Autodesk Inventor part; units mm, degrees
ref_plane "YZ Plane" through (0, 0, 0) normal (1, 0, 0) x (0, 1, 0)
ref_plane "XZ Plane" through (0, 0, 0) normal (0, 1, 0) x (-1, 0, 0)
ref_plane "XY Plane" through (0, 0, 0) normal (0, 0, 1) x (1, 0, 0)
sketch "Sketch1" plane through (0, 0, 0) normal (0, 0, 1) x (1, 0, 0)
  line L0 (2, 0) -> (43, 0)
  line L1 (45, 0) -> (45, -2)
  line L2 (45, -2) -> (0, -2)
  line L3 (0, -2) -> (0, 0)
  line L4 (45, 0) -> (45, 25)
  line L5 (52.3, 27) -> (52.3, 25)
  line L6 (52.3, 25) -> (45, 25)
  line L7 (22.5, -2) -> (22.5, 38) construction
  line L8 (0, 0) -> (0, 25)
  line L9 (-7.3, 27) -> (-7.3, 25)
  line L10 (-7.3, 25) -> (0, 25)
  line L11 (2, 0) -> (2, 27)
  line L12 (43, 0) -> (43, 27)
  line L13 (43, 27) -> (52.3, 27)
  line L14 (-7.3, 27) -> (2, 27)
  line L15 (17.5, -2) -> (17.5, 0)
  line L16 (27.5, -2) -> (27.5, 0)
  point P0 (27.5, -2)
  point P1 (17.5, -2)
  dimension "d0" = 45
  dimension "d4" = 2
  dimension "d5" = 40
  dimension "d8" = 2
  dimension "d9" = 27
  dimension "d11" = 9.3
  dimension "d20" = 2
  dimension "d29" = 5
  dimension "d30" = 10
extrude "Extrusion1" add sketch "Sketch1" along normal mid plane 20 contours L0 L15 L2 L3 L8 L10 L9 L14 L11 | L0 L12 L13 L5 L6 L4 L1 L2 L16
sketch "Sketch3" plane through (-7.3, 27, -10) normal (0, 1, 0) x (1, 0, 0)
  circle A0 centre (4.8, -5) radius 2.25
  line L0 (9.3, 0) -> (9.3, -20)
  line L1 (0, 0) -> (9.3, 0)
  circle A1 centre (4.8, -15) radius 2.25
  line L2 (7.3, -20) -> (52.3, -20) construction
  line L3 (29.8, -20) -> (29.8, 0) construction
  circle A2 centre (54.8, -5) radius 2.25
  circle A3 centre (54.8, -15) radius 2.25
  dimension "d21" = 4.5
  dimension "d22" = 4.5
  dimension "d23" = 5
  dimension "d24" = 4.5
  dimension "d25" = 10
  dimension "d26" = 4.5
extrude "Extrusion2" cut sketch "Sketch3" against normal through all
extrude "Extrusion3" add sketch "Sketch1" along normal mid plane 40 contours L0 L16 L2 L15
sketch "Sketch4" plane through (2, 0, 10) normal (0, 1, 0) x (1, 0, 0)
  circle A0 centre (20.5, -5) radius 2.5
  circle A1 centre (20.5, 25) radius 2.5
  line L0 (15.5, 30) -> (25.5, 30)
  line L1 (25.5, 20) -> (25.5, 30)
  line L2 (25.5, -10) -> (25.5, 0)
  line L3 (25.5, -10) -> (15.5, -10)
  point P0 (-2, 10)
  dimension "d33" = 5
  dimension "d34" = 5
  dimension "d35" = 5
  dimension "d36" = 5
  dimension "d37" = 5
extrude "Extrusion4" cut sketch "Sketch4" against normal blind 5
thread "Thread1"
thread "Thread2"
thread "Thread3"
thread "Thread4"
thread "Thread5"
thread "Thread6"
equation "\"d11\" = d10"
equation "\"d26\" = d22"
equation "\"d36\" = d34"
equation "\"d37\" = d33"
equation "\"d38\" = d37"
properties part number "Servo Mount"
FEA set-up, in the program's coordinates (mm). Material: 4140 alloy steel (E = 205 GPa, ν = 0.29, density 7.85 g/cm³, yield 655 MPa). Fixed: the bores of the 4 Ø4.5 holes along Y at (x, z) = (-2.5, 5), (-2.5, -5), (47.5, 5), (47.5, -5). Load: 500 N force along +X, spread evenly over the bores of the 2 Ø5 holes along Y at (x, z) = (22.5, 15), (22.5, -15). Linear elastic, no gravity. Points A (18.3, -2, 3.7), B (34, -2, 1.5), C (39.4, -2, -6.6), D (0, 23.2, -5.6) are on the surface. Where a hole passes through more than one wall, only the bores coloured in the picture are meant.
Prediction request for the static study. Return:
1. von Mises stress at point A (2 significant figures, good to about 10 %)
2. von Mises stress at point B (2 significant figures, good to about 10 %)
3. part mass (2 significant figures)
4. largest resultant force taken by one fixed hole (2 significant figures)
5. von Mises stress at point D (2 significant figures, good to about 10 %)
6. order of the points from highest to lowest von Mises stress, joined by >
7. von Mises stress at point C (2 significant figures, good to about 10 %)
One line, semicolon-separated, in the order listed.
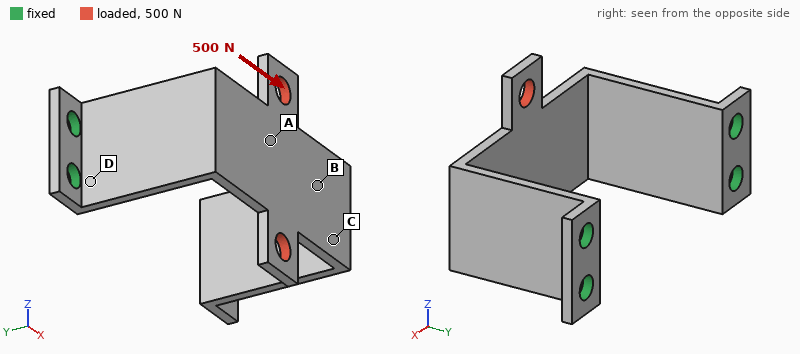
43 MPa; 99 MPa; 37 g; 140 N; 210 MPa; D > C > B > A; 150 MPa
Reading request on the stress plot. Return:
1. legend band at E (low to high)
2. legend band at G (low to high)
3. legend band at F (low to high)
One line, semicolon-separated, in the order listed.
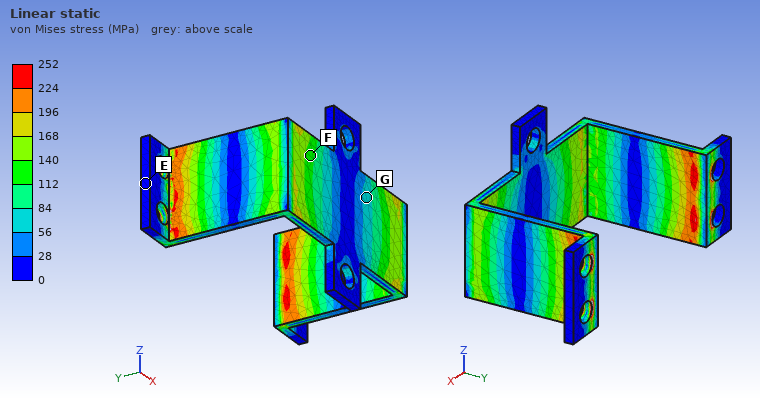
0 to 28 MPa; 56 to 84 MPa; 112 to 140 MPa
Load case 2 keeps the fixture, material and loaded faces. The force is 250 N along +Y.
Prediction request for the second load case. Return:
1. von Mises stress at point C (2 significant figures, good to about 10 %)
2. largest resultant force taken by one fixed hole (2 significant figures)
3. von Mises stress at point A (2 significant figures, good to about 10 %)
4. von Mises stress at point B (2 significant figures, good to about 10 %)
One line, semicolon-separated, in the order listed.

42 MPa; 69 N; 100 MPa; 45 MPa
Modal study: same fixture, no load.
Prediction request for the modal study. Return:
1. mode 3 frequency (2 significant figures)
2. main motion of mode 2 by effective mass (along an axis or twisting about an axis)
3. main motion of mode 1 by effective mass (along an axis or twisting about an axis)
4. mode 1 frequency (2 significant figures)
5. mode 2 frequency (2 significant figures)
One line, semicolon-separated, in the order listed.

4100 Hz; along Y; along X; 1500 Hz; 3300 Hz
